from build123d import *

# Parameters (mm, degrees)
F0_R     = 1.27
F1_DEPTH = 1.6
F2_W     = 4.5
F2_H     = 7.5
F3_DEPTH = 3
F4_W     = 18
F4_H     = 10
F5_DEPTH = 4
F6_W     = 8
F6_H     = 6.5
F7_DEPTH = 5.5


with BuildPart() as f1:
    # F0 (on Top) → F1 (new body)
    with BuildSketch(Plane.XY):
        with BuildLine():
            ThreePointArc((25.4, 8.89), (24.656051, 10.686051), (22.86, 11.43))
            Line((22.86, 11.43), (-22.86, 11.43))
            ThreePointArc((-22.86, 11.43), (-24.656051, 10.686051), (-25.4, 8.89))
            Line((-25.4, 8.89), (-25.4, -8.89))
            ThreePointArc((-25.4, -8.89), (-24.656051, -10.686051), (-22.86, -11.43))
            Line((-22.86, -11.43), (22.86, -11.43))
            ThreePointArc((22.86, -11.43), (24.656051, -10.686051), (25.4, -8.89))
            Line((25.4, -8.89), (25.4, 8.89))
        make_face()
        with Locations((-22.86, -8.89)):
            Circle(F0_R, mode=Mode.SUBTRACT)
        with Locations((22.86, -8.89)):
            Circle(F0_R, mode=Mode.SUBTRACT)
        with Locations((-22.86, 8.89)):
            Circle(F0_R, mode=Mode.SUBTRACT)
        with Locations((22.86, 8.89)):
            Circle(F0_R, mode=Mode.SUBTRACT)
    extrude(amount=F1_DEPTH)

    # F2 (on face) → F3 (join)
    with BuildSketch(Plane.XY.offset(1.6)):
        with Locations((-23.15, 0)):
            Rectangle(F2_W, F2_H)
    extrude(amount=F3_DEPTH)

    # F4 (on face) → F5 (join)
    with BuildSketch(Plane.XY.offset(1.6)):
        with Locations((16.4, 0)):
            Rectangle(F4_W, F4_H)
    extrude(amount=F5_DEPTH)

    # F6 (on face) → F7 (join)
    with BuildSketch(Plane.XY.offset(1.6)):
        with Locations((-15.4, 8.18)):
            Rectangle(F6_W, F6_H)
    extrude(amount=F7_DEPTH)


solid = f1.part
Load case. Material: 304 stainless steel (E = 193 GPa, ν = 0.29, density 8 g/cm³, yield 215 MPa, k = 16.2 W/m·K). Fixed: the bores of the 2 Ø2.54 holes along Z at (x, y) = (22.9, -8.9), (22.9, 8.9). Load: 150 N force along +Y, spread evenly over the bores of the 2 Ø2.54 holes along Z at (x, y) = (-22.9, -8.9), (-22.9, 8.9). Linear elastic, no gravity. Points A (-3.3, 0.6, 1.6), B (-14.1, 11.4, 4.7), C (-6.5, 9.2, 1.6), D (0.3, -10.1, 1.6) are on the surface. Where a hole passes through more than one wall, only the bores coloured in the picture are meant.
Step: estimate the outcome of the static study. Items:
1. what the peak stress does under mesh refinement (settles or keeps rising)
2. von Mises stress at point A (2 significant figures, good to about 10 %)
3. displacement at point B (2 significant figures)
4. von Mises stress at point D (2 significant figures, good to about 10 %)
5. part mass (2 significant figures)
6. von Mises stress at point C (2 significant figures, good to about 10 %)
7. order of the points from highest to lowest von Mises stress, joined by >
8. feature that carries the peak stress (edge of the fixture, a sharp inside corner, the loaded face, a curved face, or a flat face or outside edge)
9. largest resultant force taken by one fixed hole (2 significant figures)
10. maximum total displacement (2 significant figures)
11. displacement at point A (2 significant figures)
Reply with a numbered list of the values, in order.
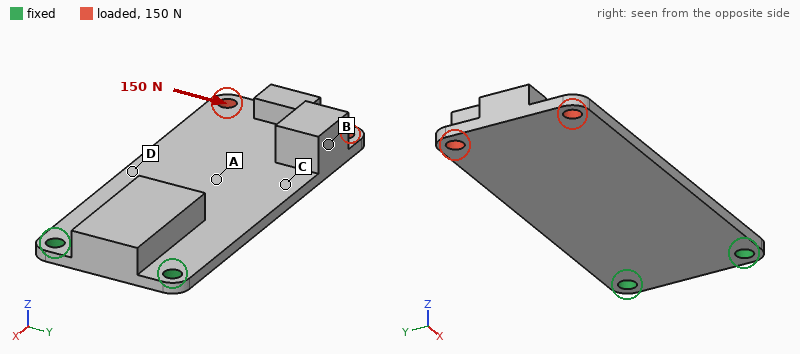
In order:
1. keeps rising
2. 10 MPa
3. 14 µm
4. 22 MPa
5. 23 g
6. 15 MPa
7. D > C > A > B
8. edge of the fixture
9. 380 N
10. 20 µm
11. 7.2 µm
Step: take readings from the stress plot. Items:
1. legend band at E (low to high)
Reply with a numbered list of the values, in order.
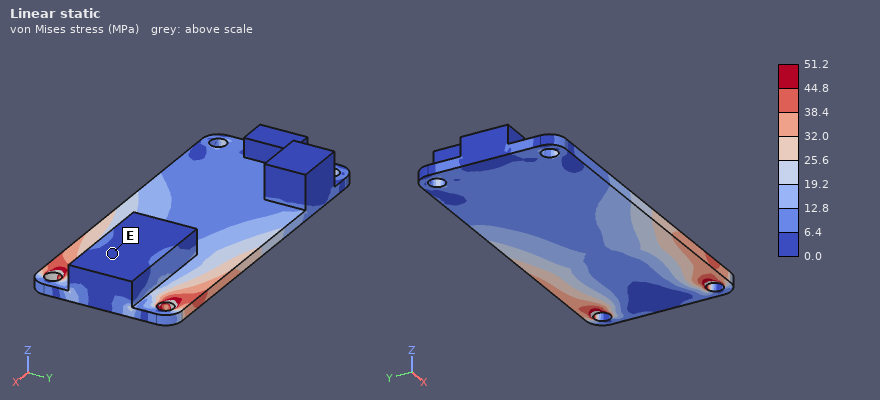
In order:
1. 0.0 to 6.4 MPa
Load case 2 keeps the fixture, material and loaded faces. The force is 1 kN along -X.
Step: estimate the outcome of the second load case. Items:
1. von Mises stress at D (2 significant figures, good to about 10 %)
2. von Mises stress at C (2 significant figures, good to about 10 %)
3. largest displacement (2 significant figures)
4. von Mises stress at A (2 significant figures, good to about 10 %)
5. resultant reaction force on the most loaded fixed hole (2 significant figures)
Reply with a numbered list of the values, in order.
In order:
1. 26 MPa
2. 30 MPa
3. 18 µm
4. 25 MPa
5. 510 N
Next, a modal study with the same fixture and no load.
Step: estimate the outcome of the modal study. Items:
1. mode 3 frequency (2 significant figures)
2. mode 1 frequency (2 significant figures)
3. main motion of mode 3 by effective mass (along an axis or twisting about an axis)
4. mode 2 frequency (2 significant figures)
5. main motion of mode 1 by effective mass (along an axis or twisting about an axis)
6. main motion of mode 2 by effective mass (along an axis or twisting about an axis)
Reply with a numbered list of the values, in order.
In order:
1. 3300 Hz
2. 650 Hz
3. along Z
4. 2700 Hz
5. along Z
6. twisting about X
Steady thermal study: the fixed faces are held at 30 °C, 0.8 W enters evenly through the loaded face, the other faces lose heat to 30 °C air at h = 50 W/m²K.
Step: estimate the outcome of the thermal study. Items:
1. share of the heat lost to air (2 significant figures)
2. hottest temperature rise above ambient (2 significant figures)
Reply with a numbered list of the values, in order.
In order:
1. 92 %
2. 22 K
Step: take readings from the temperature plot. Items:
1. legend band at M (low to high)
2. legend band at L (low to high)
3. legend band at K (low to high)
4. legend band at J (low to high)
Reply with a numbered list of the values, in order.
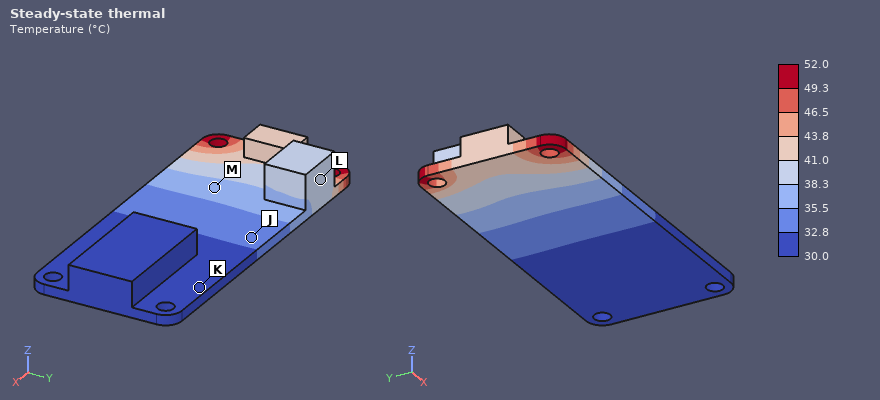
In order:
1. 35.5 to 38.3 °C
2. 38.3 to 41.0 °C
3. 30.0 to 32.8 °C
4. 32.8 to 35.5 °C
